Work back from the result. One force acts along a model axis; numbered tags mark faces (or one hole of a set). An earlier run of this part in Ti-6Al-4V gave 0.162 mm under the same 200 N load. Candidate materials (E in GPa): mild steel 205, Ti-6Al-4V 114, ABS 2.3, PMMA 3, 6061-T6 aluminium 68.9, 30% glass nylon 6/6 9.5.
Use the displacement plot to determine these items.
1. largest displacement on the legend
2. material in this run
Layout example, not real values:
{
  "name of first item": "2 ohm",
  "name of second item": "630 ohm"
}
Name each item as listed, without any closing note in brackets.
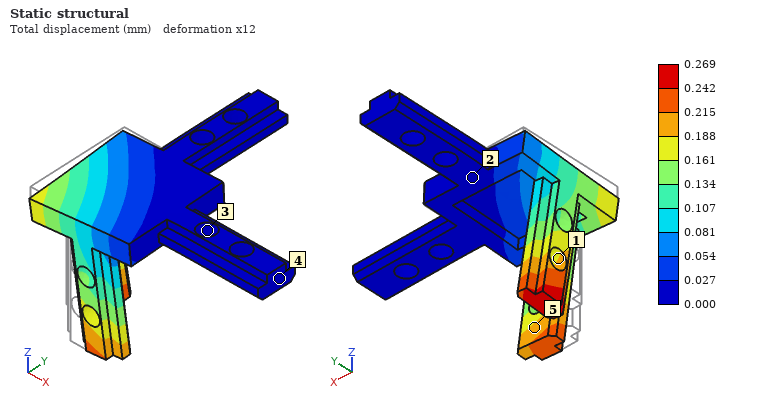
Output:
{
  "largest displacement on the legend": "0.269 mm",
  "material in this run": "6061-T6 aluminium"
}
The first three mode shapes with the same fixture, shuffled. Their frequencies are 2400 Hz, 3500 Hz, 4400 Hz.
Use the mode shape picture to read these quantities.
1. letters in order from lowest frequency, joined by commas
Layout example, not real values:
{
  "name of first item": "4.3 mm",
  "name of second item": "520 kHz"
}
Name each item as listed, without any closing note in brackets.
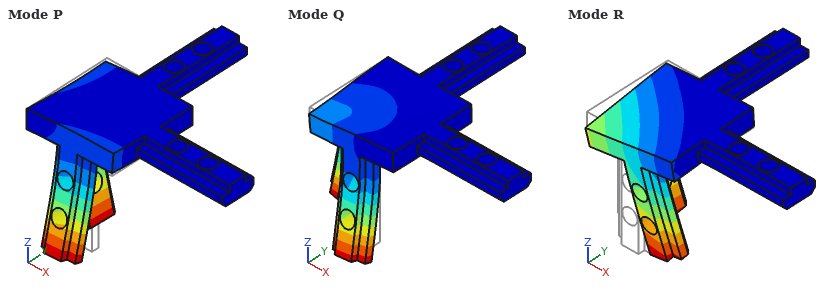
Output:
{
  "letters in order from lowest frequency, joined by commas": "R, P, Q"
}
